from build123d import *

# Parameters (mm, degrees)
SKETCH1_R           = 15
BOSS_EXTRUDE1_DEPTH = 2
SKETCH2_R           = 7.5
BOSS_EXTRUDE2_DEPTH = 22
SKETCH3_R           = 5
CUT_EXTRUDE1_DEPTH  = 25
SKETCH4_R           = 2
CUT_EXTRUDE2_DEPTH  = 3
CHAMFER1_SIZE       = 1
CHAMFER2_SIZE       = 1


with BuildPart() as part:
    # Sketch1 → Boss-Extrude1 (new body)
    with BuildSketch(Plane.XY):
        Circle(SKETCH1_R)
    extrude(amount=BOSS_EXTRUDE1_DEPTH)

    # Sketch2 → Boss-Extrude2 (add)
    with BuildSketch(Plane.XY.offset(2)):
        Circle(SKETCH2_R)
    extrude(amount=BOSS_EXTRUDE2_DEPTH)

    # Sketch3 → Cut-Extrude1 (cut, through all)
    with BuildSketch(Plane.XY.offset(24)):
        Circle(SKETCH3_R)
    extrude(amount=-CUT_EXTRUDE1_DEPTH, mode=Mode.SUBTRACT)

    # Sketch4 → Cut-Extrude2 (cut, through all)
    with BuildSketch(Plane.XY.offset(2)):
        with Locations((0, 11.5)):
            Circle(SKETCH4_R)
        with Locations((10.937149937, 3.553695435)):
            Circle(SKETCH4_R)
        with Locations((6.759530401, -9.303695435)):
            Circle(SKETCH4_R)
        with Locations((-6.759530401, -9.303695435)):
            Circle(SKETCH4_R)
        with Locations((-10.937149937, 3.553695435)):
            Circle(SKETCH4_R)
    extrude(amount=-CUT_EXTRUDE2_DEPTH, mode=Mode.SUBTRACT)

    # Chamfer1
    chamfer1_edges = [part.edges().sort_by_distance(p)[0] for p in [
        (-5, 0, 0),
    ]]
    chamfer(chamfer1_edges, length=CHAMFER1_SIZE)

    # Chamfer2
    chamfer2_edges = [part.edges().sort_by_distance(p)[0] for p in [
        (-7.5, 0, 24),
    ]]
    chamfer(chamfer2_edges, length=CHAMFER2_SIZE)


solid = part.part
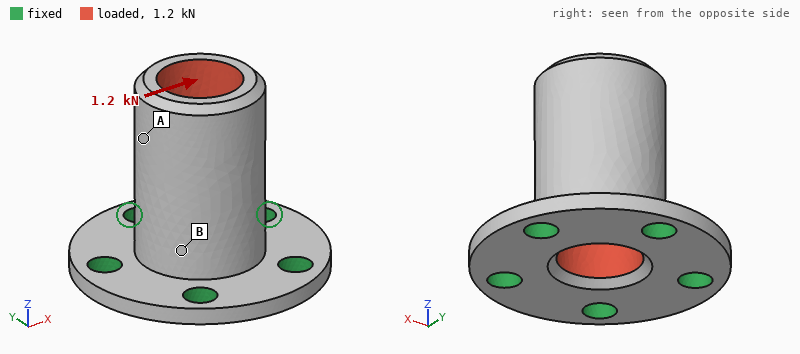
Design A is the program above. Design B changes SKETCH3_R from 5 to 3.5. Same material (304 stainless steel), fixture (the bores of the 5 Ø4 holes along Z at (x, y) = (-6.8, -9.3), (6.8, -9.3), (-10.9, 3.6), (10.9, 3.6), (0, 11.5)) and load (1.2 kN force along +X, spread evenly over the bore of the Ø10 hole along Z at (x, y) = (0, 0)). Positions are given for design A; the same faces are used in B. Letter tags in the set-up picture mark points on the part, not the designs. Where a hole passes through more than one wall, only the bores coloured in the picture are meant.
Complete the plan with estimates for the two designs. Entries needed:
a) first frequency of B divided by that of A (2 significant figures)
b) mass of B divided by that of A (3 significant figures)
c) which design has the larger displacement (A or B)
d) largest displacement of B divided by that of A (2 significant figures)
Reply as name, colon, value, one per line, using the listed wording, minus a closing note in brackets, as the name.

first frequency of B divided by that of A: 0.91
mass of B divided by that of A: 1.30
which design has the larger displacement: A
largest displacement of B divided by that of A: 0.87
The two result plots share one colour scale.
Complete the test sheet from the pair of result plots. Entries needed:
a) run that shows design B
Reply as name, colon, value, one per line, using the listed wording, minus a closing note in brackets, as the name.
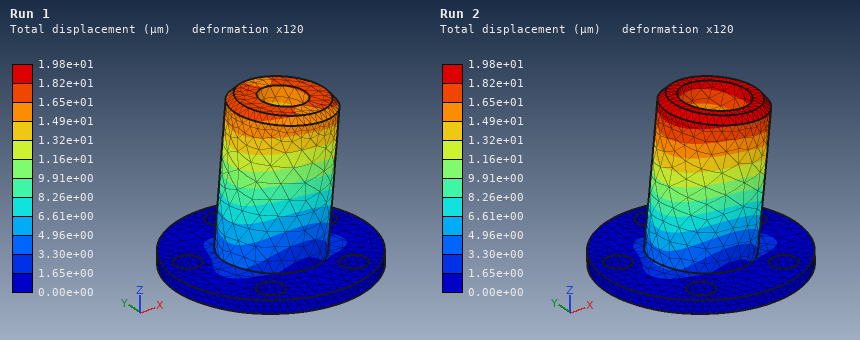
run that shows design B: Run 1
